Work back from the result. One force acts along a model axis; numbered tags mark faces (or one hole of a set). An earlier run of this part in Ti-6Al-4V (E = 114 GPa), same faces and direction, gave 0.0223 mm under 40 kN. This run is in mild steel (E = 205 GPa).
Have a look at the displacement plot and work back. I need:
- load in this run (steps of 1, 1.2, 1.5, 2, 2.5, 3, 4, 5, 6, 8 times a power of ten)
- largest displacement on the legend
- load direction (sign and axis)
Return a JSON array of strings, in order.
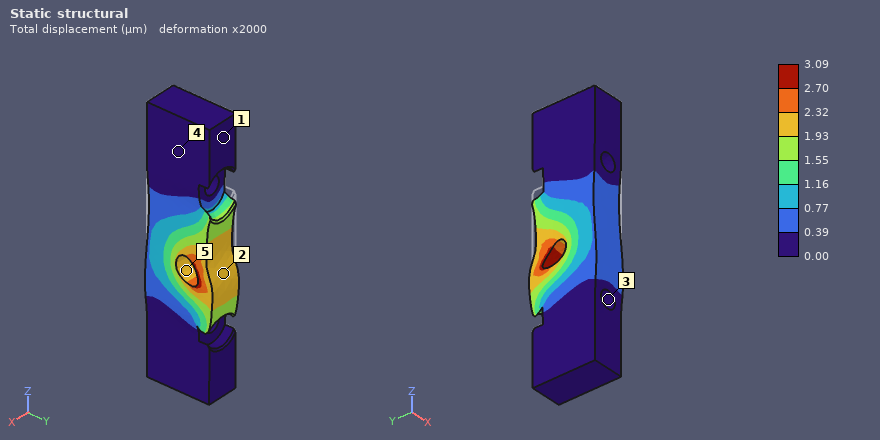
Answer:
["10 kN", "3.09 µm", "-Z"]
